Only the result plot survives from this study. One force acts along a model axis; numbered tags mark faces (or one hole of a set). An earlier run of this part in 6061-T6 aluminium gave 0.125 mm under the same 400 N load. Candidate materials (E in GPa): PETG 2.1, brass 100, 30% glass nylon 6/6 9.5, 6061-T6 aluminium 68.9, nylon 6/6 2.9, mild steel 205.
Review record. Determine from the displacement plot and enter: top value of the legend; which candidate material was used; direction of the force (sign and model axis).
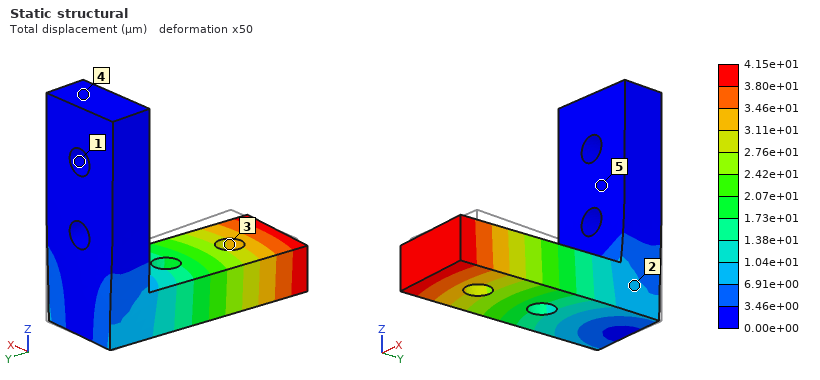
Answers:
4.15e+01 µm
mild steel
-X
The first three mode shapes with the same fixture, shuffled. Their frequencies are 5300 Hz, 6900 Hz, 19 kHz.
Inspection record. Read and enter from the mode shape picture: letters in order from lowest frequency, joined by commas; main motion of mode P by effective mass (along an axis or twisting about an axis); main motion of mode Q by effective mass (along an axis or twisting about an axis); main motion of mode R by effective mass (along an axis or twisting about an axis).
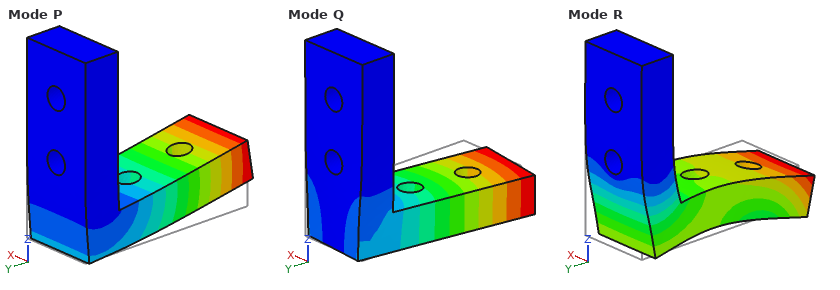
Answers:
P, Q, R
along Z
along X
along Y
